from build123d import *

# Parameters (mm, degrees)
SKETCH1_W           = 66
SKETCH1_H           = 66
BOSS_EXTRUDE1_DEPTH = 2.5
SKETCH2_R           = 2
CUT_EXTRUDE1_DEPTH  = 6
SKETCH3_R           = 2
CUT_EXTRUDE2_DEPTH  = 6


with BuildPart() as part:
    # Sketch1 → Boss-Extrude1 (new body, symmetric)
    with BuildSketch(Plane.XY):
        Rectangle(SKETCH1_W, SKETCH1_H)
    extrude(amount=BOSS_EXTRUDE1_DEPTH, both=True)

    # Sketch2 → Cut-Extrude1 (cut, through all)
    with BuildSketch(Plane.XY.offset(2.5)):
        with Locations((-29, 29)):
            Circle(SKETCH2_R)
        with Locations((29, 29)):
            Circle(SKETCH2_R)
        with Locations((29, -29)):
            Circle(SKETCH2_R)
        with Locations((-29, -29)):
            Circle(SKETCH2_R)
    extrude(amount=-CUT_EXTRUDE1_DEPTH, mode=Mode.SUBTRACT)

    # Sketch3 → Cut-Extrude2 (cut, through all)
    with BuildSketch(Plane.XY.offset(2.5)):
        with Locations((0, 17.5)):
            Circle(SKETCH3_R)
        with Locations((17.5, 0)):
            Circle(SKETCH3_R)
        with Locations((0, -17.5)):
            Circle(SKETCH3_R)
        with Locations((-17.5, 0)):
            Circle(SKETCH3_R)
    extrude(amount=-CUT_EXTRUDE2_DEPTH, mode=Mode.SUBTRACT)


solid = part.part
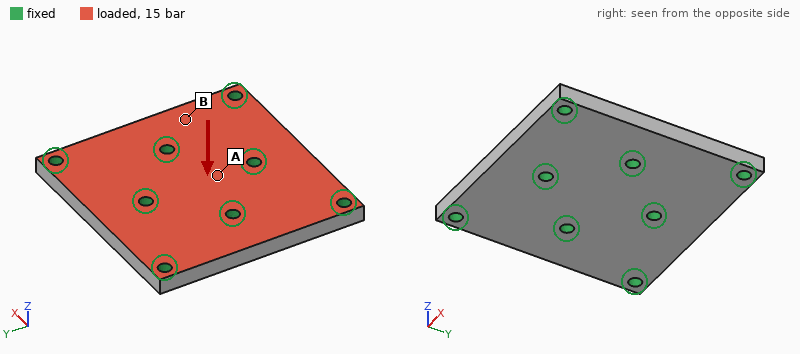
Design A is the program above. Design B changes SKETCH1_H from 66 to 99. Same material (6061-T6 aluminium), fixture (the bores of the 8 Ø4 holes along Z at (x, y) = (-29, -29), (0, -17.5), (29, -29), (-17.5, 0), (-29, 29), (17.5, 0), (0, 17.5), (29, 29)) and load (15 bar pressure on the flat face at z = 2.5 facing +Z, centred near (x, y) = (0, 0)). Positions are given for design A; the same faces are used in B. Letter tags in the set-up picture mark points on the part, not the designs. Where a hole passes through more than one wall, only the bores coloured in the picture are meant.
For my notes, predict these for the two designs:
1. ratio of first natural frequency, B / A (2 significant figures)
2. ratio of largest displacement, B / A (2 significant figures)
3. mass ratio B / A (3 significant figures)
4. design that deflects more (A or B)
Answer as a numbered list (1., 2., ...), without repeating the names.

1. 0.35
2. 10
3. 1.51
4. B
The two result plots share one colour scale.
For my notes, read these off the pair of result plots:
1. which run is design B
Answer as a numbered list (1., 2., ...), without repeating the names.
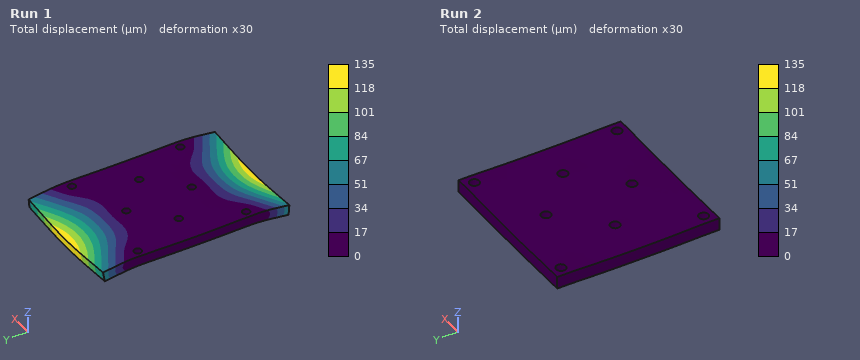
1. Run 1
